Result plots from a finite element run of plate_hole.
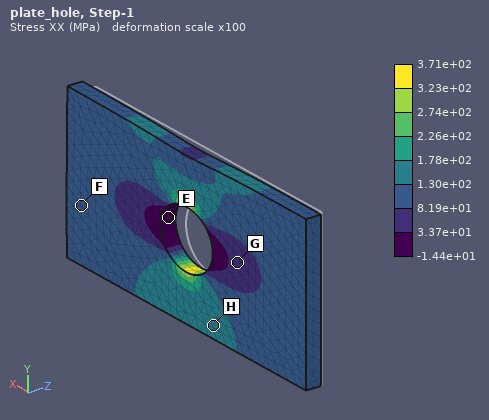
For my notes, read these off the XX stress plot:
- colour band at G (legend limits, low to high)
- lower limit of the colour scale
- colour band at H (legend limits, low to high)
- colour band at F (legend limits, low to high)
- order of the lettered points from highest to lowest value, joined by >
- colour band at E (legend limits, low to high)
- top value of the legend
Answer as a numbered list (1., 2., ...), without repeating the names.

1. 3.37e+01 to 8.19e+01 MPa
2. -1.44e+01 MPa
3. 1.30e+02 to 1.78e+02 MPa
4. 8.19e+01 to 1.30e+02 MPa
5. H > F > G > E
6. -1.44e+01 to 3.37e+01 MPa
7. 3.71e+02 MPa
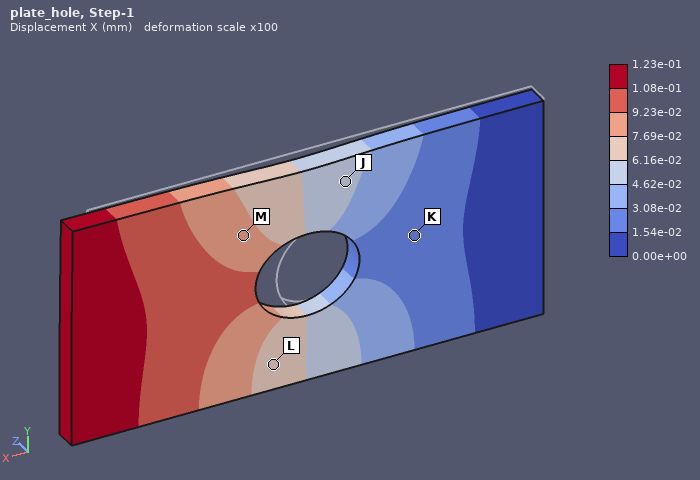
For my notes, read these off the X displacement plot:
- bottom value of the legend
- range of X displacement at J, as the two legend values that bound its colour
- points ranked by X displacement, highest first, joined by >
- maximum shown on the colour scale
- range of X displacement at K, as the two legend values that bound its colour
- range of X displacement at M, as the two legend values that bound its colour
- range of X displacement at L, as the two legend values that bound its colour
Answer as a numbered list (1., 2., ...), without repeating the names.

1. 0.00e+00 mm
2. 4.62e-02 to 6.16e-02 mm
3. M > L > J > K
4. 1.23e-01 mm
5. 1.54e-02 to 3.08e-02 mm
6. 7.69e-02 to 9.23e-02 mm
7. 6.16e-02 to 7.69e-02 mm
